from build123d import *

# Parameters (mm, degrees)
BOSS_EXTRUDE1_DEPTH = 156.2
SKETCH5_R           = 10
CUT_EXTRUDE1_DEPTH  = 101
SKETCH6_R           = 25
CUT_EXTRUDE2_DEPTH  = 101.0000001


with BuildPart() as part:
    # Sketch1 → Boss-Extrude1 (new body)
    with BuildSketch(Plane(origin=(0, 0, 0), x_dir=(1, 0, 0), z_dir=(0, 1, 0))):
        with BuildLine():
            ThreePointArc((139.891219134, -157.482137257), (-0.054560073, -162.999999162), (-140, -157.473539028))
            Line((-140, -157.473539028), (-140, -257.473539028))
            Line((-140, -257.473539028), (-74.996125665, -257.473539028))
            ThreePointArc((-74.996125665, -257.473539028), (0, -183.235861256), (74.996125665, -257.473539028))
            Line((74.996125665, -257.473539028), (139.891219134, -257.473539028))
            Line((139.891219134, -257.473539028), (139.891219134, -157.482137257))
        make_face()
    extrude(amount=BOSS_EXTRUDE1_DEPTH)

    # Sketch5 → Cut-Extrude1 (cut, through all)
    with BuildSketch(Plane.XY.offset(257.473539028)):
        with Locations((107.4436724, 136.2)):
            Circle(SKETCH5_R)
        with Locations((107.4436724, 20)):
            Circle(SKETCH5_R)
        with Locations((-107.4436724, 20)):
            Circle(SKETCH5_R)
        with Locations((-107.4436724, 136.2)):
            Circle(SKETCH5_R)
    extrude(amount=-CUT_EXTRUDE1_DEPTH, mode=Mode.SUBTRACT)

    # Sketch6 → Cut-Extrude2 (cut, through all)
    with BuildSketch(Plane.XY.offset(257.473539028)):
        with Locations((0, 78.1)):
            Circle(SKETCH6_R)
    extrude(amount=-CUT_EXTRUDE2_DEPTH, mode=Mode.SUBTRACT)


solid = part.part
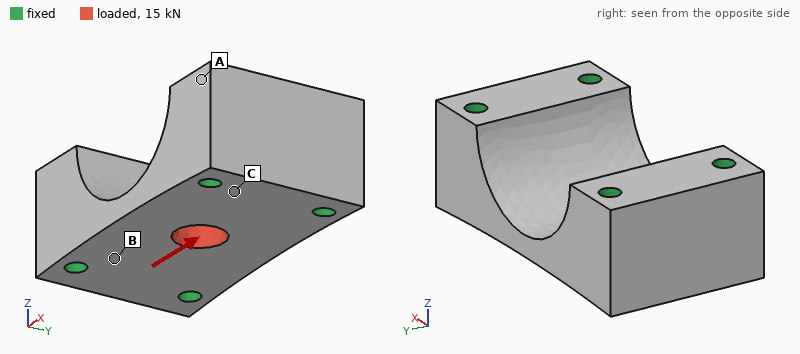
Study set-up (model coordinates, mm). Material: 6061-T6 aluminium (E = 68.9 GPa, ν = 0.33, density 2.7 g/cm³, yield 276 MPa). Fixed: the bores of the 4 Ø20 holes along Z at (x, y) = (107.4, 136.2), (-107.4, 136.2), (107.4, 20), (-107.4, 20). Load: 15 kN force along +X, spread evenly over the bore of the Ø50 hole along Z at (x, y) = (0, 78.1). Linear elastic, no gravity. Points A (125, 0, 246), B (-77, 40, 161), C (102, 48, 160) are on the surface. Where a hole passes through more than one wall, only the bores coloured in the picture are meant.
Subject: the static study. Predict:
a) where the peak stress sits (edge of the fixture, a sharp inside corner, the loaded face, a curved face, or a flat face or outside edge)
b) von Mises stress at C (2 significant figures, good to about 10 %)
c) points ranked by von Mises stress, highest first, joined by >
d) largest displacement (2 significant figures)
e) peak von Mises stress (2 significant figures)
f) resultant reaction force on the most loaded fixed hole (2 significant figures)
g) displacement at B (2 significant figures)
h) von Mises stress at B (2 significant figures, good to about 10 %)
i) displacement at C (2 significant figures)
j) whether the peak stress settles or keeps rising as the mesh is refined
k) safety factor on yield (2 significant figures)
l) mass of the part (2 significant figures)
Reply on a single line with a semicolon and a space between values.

the loaded face; 1.2 MPa; B > C > A; 4.4 µm; 8.7 MPa; 3.9 kN; 1.0 µm; 2.2 MPa; 0.80 µm; settles; 32; 7.2 kg
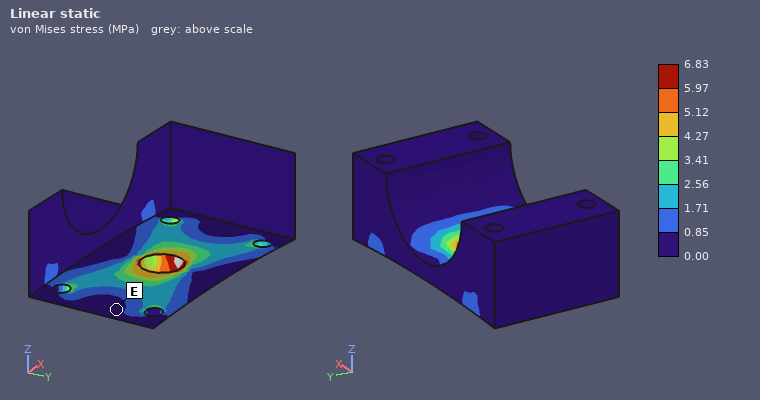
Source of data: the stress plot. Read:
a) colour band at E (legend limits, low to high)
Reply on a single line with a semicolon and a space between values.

0.00 to 0.85 MPa
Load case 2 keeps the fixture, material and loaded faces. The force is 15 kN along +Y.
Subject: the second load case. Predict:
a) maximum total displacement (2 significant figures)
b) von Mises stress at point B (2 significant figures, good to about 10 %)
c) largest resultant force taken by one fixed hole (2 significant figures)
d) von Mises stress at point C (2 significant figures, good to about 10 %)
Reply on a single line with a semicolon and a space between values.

7.0 µm; 2.3 MPa; 5.7 kN; 1.2 MPa
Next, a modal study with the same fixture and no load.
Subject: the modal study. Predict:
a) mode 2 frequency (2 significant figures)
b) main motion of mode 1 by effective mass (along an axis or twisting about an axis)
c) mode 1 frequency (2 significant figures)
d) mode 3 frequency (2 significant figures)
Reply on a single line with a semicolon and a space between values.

7700 Hz; along Z; 6700 Hz; 8600 Hz
